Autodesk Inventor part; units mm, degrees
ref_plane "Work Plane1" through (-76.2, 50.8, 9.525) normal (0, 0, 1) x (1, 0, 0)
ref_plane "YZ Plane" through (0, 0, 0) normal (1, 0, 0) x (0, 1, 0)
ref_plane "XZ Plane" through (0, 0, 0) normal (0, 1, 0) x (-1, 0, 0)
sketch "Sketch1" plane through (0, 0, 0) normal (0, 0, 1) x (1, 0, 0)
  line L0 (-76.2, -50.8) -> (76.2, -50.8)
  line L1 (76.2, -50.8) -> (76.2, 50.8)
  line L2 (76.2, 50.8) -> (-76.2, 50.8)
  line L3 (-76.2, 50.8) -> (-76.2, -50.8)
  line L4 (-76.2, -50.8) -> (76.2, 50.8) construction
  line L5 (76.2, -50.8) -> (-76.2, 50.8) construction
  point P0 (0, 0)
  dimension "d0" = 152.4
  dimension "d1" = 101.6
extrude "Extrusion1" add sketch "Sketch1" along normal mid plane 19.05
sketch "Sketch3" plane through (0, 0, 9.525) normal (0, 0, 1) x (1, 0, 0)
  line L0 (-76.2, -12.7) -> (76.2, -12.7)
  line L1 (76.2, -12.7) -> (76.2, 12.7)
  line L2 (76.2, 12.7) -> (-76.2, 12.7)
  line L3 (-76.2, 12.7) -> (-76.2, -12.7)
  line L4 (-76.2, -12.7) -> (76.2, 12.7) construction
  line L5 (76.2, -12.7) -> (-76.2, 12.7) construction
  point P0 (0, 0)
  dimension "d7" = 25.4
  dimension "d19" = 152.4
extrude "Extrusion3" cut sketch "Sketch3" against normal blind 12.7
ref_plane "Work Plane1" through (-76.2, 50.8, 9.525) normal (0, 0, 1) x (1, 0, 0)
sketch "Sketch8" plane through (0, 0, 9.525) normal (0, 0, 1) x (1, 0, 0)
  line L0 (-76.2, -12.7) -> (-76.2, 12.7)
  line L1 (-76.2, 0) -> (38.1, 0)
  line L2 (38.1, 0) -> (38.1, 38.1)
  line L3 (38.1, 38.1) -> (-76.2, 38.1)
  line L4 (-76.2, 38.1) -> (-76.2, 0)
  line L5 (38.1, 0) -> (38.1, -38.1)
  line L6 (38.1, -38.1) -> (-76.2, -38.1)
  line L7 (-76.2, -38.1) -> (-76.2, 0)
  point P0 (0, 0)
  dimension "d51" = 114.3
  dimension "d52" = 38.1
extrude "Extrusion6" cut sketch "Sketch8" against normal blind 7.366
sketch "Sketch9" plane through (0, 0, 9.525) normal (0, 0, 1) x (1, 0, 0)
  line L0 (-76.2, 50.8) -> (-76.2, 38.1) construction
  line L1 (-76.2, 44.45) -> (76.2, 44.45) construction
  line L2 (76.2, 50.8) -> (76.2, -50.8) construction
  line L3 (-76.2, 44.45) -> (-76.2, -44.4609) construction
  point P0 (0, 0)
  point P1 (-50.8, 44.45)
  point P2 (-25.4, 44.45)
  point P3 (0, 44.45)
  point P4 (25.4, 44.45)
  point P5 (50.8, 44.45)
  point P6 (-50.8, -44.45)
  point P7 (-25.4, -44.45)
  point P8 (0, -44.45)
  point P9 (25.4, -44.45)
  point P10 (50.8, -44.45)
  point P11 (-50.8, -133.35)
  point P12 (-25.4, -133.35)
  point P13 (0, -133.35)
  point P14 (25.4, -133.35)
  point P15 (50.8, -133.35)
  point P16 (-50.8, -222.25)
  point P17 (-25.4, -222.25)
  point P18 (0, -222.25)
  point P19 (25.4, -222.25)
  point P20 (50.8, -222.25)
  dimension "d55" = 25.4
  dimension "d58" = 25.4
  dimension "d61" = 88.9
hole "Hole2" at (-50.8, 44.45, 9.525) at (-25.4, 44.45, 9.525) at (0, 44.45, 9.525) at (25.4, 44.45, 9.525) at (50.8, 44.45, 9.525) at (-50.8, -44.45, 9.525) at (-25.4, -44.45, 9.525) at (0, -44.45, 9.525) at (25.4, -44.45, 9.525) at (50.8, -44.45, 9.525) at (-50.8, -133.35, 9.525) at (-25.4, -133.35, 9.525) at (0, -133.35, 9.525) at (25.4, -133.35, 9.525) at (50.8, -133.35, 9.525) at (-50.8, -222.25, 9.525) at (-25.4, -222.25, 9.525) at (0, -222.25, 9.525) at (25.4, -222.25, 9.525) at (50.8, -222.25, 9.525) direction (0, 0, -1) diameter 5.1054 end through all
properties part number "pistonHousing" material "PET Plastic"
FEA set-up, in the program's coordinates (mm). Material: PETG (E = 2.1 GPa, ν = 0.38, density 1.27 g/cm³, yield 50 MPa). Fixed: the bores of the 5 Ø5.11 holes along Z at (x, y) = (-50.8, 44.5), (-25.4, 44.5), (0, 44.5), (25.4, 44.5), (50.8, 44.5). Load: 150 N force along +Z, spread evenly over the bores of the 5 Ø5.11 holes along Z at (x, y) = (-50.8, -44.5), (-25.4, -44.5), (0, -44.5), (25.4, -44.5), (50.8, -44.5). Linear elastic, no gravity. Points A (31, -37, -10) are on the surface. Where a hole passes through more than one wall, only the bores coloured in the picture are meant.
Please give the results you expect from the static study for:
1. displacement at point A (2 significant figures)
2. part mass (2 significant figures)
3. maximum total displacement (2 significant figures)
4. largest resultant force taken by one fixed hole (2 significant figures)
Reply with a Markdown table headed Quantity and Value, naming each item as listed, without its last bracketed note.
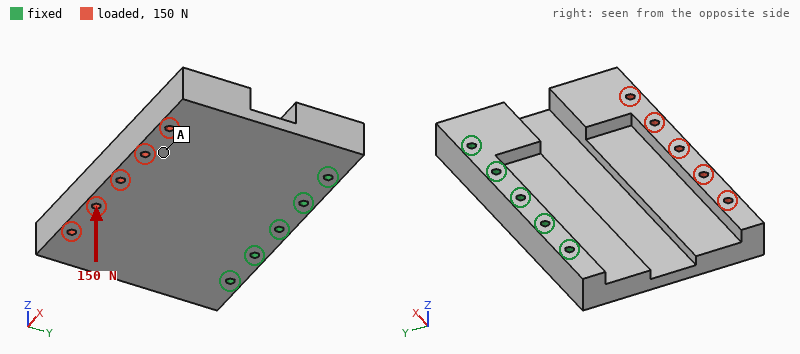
| Quantity | Value |
|---|---|
| displacement at point A | 1.4 mm |
| part mass | 250 g |
| maximum total displacement | 1.9 mm |
| largest resultant force taken by one fixed hole | 48 N |
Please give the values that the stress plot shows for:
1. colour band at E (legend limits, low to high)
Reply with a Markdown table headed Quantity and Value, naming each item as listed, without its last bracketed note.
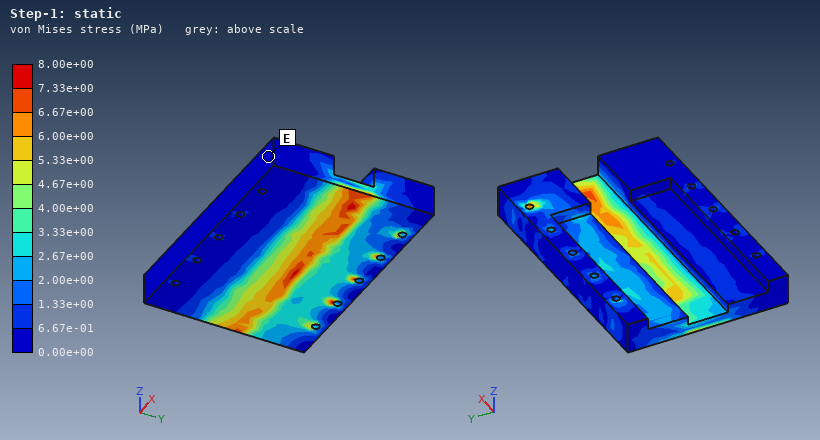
| Quantity | Value |
|---|---|
| colour band at E | 0.00e+00 to 6.67e-01 MPa |
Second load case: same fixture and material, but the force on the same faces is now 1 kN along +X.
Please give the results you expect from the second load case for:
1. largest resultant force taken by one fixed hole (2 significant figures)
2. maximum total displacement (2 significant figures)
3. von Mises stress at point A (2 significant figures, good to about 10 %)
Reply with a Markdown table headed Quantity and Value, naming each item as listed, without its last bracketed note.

| Quantity | Value |
|---|---|
| largest resultant force taken by one fixed hole | 800 N |
| maximum total displacement | 0.51 mm |
| von Mises stress at point A | 0.66 MPa |
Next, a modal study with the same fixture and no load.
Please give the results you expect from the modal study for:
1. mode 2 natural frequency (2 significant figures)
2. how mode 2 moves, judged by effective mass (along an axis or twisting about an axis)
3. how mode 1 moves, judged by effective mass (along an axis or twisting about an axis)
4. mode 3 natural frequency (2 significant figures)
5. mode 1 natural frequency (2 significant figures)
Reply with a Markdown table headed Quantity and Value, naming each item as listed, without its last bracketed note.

| Quantity | Value |
|---|---|
| mode 2 natural frequency | 370 Hz |
| how mode 2 moves, judged by effective mass | twisting about Y |
| how mode 1 moves, judged by effective mass | along Z |
| mode 3 natural frequency | 990 Hz |
| mode 1 natural frequency | 180 Hz |
